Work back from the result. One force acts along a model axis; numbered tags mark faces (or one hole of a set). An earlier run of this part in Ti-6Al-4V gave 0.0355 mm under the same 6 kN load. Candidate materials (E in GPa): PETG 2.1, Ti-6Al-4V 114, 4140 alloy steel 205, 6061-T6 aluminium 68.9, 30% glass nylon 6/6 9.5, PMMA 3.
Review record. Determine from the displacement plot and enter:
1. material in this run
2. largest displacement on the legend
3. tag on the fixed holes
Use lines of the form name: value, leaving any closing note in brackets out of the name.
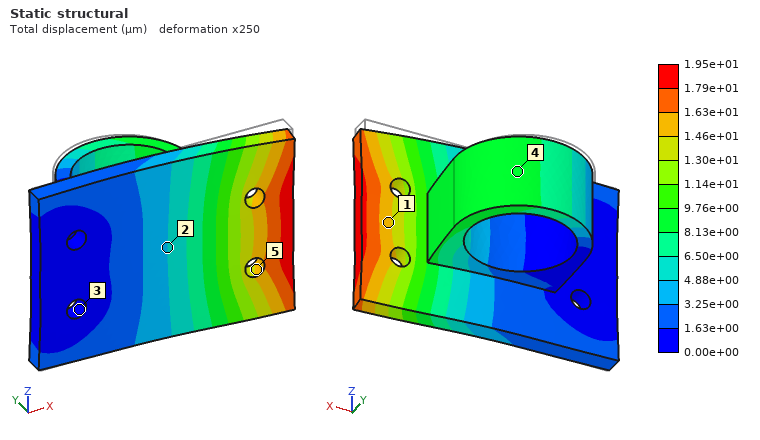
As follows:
material in this run: 4140 alloy steel
largest displacement on the legend: 1.95e+01 µm
tag on the fixed holes: 3
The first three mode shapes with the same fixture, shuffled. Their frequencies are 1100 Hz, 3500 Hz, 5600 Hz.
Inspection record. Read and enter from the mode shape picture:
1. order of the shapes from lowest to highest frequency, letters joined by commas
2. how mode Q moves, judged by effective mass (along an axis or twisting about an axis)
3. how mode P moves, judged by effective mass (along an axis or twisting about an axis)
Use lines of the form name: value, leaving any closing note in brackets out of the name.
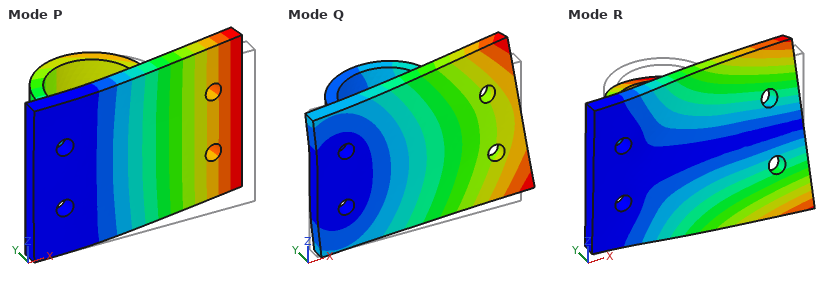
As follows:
order of the shapes from lowest to highest frequency, letters joined by commas: P, R, Q
how mode Q moves, judged by effective mass: along Z
how mode P moves, judged by effective mass: along Y
